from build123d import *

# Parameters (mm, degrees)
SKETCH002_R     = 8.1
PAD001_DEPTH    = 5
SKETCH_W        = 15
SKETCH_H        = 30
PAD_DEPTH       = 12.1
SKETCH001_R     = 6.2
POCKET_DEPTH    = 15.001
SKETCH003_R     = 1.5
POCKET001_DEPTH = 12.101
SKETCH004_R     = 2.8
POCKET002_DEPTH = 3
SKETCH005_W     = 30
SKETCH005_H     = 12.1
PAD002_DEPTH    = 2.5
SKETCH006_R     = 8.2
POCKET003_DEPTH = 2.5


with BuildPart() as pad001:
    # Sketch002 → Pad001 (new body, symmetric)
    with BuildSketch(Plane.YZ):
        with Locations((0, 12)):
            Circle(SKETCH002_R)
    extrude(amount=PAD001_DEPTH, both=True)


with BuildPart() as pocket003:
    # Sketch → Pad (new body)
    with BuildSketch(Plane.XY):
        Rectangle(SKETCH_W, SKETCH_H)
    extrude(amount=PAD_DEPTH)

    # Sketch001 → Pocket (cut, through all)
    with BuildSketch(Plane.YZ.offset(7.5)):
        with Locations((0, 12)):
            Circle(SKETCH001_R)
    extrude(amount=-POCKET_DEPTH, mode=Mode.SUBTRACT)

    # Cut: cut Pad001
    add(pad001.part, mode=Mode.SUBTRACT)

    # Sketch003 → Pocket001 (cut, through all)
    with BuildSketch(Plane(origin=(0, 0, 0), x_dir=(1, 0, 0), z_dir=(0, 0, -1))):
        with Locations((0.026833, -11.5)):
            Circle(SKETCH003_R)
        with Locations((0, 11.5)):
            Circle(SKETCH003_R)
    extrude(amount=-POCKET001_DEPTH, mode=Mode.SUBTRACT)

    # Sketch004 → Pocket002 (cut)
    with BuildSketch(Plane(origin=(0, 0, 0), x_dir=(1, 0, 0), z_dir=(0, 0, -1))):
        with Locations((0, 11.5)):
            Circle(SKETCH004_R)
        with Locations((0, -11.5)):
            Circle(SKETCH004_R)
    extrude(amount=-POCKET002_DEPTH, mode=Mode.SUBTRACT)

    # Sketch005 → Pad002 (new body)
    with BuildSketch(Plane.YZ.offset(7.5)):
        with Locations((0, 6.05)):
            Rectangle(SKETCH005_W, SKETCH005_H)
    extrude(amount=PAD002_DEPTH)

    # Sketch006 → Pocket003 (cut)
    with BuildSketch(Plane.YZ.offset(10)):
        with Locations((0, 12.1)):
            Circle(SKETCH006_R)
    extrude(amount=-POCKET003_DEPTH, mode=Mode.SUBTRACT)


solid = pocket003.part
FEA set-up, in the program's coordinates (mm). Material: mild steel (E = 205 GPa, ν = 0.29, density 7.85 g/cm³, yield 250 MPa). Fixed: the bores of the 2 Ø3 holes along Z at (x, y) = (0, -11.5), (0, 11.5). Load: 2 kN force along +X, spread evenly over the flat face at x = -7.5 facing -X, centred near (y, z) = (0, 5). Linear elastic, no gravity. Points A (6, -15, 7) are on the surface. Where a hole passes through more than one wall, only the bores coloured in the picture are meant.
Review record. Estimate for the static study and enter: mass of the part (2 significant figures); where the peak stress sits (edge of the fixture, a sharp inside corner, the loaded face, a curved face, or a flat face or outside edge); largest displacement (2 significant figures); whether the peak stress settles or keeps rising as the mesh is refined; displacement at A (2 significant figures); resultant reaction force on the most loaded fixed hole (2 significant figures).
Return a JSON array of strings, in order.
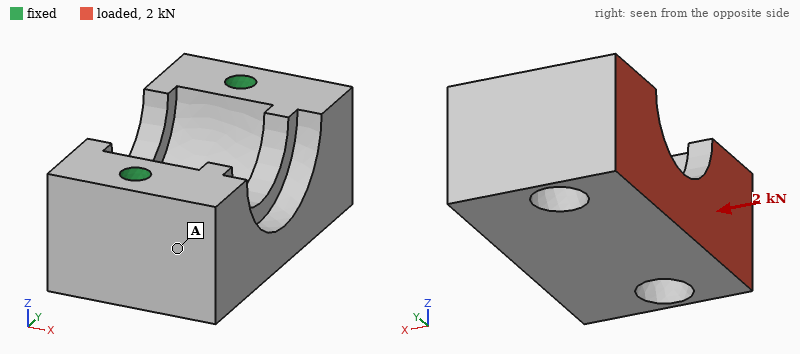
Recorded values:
["35 g", "edge of the fixture", "1.3 µm", "keeps rising", "0.25 µm", "1.0 kN"]
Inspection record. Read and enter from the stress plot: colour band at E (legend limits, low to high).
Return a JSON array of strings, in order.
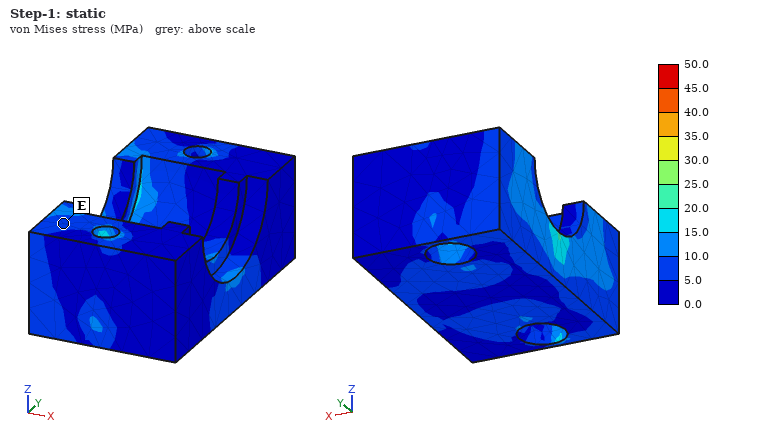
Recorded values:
["5.0 to 10.0 MPa"]
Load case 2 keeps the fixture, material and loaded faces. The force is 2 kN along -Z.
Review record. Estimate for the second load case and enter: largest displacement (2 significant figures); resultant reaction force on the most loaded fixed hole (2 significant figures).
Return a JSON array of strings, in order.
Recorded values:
["4.2 µm", "1.0 kN"]
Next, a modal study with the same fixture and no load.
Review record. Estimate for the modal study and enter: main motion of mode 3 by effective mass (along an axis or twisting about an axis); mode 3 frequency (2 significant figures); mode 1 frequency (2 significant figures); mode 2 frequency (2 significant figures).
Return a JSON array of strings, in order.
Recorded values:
["along Z", "47 kHz", "33 kHz", "44 kHz"]
